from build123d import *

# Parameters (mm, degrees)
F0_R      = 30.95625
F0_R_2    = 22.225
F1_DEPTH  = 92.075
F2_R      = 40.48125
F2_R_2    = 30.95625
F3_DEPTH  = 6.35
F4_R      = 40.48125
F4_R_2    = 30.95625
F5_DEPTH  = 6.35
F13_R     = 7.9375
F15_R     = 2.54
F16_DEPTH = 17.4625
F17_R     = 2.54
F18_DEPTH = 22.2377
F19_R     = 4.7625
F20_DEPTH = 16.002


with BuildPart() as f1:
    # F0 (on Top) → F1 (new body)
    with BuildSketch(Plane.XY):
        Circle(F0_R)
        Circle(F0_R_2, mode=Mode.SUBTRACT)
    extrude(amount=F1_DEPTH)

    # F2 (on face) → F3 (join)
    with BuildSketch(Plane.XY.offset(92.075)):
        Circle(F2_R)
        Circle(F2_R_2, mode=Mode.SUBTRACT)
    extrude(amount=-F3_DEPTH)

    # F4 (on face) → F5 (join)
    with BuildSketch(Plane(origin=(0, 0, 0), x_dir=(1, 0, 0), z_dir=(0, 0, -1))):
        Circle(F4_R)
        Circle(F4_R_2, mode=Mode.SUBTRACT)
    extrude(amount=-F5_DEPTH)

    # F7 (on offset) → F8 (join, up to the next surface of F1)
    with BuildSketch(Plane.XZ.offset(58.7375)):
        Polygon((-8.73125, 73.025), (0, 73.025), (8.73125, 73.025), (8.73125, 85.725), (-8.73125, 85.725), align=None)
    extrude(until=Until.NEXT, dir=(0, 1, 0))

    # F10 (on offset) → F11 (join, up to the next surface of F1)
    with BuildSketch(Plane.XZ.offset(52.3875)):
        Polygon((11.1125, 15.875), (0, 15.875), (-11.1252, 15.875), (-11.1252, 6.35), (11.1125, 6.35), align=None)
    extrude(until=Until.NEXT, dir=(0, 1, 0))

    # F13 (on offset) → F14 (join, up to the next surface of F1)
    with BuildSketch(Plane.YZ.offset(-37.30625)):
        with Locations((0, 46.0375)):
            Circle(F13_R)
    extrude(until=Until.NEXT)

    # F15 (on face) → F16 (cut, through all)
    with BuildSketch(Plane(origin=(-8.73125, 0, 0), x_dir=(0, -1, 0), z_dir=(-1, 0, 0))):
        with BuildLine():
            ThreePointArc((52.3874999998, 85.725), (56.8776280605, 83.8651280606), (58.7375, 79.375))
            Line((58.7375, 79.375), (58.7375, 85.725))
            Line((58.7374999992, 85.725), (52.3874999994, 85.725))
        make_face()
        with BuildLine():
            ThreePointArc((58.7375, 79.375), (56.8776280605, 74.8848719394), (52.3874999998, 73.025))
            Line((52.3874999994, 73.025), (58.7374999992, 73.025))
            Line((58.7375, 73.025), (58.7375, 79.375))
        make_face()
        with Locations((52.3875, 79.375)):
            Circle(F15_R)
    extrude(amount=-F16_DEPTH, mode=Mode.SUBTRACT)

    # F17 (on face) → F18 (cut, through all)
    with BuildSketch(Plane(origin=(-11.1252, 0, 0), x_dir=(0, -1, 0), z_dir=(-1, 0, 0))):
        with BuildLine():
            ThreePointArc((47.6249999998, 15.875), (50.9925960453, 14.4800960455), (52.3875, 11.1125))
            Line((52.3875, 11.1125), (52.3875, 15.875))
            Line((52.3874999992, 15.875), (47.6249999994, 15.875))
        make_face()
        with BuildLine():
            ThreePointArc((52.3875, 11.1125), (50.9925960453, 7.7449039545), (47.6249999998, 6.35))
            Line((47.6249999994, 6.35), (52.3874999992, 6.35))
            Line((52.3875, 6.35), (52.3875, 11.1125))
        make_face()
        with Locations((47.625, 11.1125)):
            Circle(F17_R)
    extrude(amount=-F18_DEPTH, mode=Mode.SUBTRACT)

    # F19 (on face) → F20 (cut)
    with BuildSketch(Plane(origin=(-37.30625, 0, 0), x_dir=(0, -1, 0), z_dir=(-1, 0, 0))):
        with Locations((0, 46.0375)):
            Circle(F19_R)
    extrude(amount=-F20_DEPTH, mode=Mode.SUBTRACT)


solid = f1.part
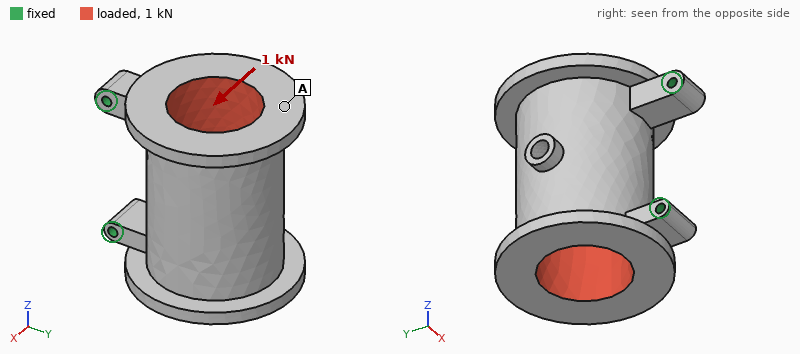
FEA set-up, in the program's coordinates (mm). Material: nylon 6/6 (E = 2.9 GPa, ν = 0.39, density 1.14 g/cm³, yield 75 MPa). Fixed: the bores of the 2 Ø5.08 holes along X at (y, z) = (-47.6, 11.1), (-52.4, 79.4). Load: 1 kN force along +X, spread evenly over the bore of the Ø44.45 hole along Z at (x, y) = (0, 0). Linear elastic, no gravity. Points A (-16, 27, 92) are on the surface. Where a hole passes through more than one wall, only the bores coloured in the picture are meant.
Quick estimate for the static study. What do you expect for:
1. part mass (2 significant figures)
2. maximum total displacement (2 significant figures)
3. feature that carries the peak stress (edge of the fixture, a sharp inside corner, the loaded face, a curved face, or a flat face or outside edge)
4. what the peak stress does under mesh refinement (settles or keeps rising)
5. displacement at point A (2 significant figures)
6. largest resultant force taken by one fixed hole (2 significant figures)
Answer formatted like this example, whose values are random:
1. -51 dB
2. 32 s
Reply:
1. 200 g
2. 1.9 mm
3. edge of the fixture
4. keeps rising
5. 1.6 mm
6. 500 N
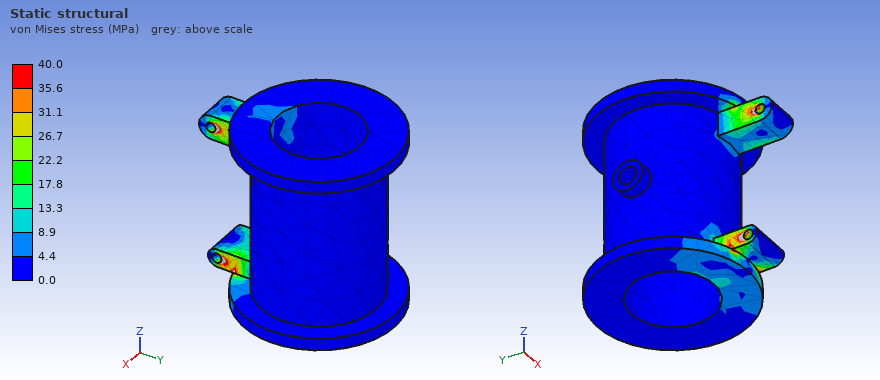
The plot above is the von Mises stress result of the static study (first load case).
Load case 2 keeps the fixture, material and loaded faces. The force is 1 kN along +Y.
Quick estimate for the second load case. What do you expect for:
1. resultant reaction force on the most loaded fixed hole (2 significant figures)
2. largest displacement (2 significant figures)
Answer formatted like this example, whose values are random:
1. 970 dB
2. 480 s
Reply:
1. 510 N
2. 76 µm
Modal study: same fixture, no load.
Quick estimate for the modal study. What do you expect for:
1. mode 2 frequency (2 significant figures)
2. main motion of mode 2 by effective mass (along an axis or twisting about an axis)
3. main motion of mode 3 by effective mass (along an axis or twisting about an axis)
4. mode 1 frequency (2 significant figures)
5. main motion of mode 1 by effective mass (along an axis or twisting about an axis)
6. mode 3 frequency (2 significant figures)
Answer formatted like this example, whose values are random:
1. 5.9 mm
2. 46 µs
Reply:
1. 770 Hz
2. along Z
3. twisting about Y
4. 320 Hz
5. along X
6. 1200 Hz
